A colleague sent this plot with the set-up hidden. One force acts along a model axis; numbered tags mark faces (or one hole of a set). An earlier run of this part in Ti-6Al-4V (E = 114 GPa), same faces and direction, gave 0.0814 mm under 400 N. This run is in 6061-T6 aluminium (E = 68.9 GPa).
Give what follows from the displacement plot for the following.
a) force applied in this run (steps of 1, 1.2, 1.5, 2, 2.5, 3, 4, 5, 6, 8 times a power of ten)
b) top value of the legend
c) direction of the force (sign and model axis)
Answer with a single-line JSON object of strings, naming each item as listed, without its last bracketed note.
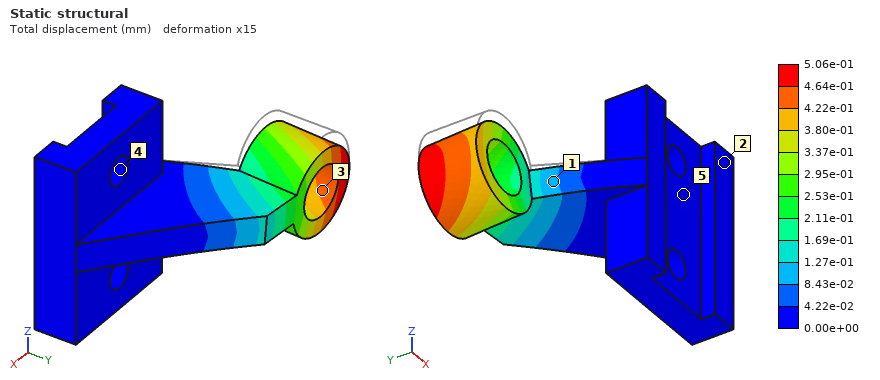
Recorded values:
{"force applied in this run": "1.5 kN", "top value of the legend": "5.06e-01 mm", "direction of the force": "-Z"}
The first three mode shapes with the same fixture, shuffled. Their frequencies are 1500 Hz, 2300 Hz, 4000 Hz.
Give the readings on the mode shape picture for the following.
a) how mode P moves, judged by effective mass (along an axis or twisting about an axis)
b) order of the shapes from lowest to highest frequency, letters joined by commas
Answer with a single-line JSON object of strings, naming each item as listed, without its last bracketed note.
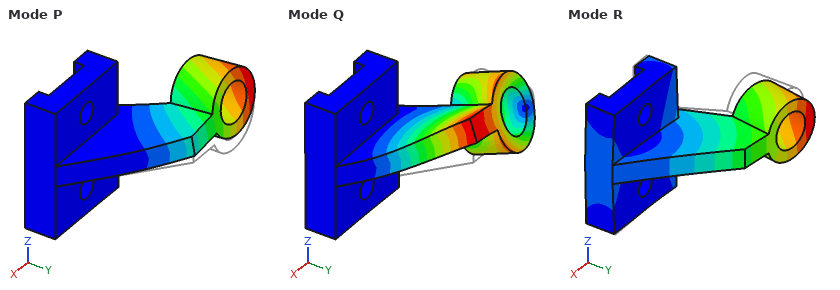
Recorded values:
{"how mode P moves, judged by effective mass": "along Z", "order of the shapes from lowest to highest frequency, letters joined by commas": "P, R, Q"}
